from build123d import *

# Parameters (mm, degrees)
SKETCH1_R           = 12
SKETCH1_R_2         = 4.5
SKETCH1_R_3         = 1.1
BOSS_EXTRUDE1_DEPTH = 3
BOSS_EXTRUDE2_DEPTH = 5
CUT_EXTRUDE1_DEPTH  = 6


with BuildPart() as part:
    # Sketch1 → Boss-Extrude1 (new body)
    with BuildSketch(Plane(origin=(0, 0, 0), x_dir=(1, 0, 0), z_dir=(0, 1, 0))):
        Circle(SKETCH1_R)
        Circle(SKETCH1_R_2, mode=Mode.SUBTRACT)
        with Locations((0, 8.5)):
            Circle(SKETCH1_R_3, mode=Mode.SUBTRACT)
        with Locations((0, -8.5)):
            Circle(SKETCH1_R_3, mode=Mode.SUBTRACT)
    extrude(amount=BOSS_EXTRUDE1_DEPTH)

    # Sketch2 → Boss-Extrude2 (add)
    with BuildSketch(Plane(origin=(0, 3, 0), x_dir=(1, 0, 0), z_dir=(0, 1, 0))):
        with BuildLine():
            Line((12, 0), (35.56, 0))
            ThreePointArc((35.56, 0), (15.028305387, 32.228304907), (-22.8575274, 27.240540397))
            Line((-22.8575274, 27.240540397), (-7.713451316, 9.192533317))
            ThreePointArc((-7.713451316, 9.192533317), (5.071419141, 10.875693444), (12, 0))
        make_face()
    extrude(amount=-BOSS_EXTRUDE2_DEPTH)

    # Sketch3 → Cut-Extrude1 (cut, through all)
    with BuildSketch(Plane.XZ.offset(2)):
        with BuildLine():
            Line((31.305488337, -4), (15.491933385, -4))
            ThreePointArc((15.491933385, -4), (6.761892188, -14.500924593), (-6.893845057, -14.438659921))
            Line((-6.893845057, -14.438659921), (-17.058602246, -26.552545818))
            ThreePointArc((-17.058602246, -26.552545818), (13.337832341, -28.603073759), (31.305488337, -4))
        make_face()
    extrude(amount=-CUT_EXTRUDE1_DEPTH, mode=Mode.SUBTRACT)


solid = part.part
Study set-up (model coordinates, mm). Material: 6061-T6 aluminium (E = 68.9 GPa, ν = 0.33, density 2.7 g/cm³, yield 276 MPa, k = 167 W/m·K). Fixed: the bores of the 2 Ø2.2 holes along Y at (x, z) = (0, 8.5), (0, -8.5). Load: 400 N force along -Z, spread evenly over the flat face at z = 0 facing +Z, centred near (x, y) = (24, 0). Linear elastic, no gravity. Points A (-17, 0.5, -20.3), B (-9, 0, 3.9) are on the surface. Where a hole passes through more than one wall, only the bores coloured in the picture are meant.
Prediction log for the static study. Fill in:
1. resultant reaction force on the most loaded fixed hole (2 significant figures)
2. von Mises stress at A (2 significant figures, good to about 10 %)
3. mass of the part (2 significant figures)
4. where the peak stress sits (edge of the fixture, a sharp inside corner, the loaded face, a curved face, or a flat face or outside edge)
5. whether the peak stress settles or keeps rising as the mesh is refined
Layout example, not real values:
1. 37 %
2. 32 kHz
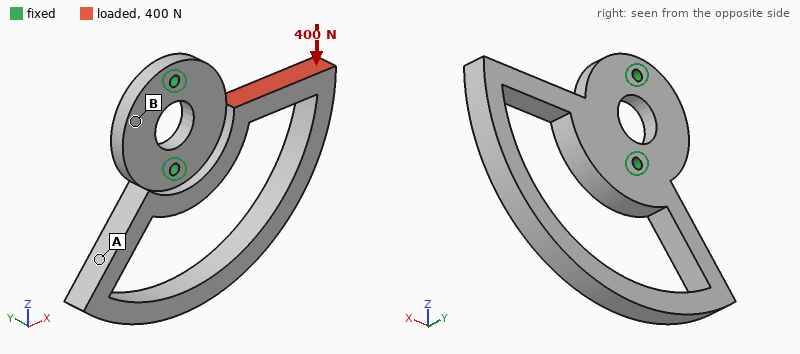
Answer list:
1. 570 N
2. 29 MPa
3. 11 g
4. a sharp inside corner
5. keeps rising
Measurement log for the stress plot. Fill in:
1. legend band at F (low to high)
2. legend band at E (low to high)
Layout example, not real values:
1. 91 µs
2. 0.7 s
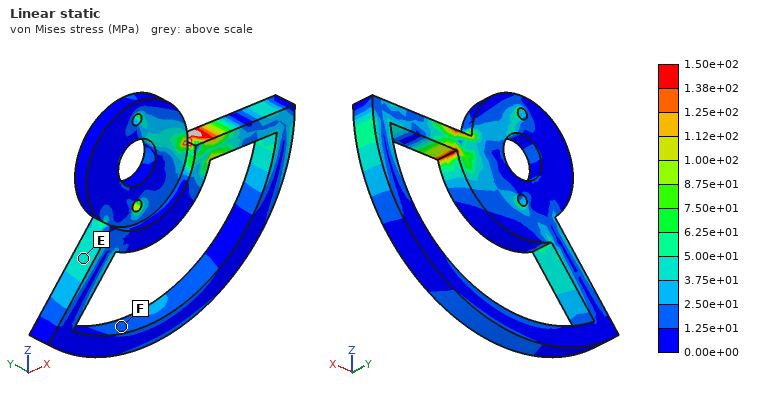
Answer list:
1. 1.25e+01 to 2.50e+01 MPa
2. 3.75e+01 to 5.00e+01 MPa
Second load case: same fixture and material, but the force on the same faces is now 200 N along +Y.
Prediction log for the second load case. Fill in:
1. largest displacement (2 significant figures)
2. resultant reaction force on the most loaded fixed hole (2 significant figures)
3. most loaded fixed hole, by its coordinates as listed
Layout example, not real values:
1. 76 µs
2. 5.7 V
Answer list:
1. 0.48 mm
2. 120 N
3. (0, -8.5)
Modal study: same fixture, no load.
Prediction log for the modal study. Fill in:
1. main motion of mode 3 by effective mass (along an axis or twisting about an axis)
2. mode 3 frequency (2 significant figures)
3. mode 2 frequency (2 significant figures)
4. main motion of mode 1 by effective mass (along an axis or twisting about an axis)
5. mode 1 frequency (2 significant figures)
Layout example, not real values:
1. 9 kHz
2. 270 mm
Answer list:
1. along X
2. 2600 Hz
3. 2200 Hz
4. along Y
5. 1400 Hz
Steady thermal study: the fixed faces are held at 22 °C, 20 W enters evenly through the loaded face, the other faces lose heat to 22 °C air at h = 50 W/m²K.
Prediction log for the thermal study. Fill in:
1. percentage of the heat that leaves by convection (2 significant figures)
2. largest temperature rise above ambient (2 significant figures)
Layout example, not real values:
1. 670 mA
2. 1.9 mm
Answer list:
1. 18 %
2. 68 K
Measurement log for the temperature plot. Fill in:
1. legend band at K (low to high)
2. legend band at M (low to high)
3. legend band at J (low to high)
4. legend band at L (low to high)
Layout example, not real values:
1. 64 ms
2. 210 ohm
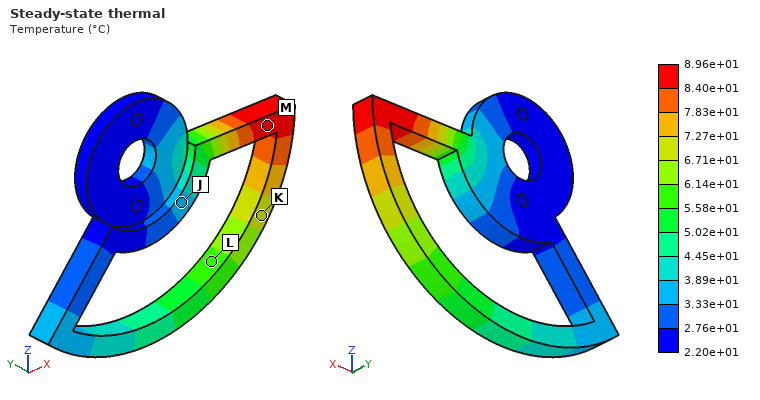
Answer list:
1. 6.71e+01 to 7.27e+01 °C
2. 8.40e+01 to 8.96e+01 °C
3. 3.33e+01 to 3.89e+01 °C
4. 5.58e+01 to 6.14e+01 °C
